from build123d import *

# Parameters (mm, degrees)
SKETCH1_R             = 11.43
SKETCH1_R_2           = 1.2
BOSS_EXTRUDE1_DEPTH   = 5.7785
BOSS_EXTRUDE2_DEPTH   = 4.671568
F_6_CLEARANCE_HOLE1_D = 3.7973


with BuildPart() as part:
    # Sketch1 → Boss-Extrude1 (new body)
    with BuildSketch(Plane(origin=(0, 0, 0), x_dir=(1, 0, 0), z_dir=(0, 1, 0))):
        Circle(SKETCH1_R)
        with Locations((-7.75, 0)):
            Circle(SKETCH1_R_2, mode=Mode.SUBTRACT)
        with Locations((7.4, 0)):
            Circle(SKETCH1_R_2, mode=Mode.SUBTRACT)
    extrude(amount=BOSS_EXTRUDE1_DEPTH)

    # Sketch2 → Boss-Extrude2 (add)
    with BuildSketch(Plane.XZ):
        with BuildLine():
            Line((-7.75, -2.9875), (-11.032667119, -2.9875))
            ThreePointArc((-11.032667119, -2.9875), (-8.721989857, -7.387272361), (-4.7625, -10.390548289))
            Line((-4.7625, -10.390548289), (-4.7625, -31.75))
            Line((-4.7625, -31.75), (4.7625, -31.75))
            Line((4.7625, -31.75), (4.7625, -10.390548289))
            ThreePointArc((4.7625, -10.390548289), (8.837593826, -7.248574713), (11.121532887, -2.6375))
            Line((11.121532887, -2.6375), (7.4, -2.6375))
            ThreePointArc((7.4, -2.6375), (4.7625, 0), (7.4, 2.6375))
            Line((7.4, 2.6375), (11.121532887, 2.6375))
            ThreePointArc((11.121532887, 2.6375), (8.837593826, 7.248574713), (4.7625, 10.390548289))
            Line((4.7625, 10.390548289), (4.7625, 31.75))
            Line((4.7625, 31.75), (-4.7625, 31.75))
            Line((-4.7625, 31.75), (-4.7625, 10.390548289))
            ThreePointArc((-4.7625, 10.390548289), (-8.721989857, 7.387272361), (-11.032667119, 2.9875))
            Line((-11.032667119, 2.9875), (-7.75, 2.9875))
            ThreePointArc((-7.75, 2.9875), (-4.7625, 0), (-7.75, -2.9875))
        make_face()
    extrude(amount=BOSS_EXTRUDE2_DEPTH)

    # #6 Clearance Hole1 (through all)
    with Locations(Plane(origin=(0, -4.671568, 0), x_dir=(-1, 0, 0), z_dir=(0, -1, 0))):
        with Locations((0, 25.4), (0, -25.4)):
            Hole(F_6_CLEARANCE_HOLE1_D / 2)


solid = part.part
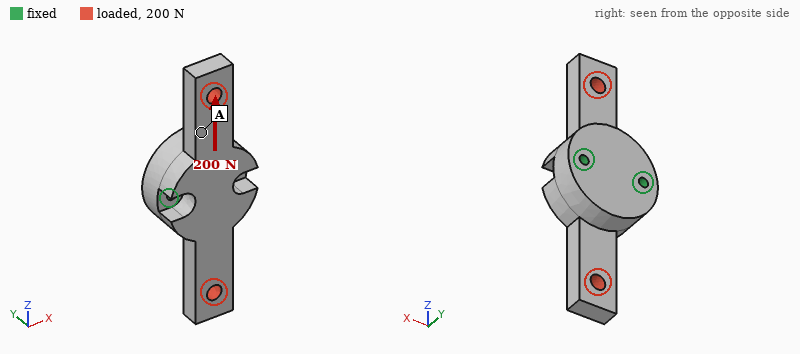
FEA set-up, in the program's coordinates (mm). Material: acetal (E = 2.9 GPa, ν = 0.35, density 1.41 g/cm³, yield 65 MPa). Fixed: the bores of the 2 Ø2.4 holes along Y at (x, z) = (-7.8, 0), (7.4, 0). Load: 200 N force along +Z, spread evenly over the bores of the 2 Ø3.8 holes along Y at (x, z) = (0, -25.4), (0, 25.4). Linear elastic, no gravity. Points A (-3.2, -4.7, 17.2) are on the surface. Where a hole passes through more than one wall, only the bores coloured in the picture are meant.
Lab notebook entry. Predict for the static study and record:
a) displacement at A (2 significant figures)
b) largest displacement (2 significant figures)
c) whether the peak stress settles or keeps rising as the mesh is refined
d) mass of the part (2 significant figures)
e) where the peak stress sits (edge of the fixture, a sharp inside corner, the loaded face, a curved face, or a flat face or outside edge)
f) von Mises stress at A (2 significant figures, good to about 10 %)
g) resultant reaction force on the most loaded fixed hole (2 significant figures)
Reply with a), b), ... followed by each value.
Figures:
a) 0.073 mm
b) 0.13 mm
c) keeps rising
d) 8.0 g
e) edge of the fixture
f) 2.2 MPa
g) 100 N
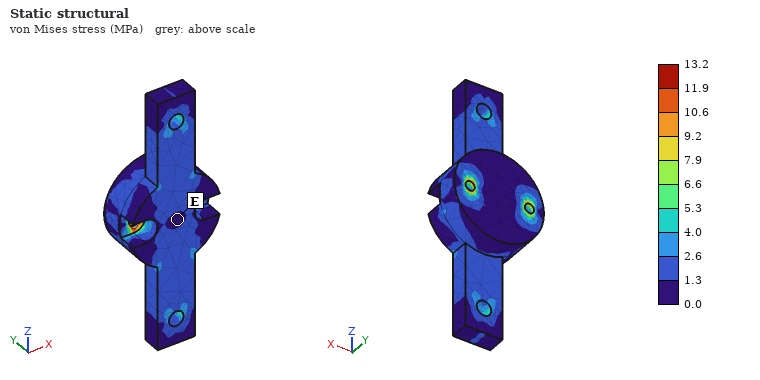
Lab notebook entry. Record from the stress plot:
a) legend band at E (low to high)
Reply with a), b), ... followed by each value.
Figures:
a) 0.0 to 1.3 MPa
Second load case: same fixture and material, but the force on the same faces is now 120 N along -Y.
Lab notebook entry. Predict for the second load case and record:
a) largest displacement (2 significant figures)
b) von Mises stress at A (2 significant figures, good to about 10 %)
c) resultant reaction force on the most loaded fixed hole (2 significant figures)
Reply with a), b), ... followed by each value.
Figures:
a) 0.68 mm
b) 14 MPa
c) 80 N
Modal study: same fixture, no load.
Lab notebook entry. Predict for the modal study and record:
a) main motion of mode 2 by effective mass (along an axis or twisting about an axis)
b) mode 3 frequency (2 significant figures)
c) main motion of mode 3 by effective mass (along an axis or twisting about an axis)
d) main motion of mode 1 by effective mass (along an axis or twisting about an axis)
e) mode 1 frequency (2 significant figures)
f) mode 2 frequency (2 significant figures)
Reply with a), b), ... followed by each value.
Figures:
a) along Y
b) 3300 Hz
c) twisting about Y
d) twisting about X
e) 1600 Hz
f) 2000 Hz
